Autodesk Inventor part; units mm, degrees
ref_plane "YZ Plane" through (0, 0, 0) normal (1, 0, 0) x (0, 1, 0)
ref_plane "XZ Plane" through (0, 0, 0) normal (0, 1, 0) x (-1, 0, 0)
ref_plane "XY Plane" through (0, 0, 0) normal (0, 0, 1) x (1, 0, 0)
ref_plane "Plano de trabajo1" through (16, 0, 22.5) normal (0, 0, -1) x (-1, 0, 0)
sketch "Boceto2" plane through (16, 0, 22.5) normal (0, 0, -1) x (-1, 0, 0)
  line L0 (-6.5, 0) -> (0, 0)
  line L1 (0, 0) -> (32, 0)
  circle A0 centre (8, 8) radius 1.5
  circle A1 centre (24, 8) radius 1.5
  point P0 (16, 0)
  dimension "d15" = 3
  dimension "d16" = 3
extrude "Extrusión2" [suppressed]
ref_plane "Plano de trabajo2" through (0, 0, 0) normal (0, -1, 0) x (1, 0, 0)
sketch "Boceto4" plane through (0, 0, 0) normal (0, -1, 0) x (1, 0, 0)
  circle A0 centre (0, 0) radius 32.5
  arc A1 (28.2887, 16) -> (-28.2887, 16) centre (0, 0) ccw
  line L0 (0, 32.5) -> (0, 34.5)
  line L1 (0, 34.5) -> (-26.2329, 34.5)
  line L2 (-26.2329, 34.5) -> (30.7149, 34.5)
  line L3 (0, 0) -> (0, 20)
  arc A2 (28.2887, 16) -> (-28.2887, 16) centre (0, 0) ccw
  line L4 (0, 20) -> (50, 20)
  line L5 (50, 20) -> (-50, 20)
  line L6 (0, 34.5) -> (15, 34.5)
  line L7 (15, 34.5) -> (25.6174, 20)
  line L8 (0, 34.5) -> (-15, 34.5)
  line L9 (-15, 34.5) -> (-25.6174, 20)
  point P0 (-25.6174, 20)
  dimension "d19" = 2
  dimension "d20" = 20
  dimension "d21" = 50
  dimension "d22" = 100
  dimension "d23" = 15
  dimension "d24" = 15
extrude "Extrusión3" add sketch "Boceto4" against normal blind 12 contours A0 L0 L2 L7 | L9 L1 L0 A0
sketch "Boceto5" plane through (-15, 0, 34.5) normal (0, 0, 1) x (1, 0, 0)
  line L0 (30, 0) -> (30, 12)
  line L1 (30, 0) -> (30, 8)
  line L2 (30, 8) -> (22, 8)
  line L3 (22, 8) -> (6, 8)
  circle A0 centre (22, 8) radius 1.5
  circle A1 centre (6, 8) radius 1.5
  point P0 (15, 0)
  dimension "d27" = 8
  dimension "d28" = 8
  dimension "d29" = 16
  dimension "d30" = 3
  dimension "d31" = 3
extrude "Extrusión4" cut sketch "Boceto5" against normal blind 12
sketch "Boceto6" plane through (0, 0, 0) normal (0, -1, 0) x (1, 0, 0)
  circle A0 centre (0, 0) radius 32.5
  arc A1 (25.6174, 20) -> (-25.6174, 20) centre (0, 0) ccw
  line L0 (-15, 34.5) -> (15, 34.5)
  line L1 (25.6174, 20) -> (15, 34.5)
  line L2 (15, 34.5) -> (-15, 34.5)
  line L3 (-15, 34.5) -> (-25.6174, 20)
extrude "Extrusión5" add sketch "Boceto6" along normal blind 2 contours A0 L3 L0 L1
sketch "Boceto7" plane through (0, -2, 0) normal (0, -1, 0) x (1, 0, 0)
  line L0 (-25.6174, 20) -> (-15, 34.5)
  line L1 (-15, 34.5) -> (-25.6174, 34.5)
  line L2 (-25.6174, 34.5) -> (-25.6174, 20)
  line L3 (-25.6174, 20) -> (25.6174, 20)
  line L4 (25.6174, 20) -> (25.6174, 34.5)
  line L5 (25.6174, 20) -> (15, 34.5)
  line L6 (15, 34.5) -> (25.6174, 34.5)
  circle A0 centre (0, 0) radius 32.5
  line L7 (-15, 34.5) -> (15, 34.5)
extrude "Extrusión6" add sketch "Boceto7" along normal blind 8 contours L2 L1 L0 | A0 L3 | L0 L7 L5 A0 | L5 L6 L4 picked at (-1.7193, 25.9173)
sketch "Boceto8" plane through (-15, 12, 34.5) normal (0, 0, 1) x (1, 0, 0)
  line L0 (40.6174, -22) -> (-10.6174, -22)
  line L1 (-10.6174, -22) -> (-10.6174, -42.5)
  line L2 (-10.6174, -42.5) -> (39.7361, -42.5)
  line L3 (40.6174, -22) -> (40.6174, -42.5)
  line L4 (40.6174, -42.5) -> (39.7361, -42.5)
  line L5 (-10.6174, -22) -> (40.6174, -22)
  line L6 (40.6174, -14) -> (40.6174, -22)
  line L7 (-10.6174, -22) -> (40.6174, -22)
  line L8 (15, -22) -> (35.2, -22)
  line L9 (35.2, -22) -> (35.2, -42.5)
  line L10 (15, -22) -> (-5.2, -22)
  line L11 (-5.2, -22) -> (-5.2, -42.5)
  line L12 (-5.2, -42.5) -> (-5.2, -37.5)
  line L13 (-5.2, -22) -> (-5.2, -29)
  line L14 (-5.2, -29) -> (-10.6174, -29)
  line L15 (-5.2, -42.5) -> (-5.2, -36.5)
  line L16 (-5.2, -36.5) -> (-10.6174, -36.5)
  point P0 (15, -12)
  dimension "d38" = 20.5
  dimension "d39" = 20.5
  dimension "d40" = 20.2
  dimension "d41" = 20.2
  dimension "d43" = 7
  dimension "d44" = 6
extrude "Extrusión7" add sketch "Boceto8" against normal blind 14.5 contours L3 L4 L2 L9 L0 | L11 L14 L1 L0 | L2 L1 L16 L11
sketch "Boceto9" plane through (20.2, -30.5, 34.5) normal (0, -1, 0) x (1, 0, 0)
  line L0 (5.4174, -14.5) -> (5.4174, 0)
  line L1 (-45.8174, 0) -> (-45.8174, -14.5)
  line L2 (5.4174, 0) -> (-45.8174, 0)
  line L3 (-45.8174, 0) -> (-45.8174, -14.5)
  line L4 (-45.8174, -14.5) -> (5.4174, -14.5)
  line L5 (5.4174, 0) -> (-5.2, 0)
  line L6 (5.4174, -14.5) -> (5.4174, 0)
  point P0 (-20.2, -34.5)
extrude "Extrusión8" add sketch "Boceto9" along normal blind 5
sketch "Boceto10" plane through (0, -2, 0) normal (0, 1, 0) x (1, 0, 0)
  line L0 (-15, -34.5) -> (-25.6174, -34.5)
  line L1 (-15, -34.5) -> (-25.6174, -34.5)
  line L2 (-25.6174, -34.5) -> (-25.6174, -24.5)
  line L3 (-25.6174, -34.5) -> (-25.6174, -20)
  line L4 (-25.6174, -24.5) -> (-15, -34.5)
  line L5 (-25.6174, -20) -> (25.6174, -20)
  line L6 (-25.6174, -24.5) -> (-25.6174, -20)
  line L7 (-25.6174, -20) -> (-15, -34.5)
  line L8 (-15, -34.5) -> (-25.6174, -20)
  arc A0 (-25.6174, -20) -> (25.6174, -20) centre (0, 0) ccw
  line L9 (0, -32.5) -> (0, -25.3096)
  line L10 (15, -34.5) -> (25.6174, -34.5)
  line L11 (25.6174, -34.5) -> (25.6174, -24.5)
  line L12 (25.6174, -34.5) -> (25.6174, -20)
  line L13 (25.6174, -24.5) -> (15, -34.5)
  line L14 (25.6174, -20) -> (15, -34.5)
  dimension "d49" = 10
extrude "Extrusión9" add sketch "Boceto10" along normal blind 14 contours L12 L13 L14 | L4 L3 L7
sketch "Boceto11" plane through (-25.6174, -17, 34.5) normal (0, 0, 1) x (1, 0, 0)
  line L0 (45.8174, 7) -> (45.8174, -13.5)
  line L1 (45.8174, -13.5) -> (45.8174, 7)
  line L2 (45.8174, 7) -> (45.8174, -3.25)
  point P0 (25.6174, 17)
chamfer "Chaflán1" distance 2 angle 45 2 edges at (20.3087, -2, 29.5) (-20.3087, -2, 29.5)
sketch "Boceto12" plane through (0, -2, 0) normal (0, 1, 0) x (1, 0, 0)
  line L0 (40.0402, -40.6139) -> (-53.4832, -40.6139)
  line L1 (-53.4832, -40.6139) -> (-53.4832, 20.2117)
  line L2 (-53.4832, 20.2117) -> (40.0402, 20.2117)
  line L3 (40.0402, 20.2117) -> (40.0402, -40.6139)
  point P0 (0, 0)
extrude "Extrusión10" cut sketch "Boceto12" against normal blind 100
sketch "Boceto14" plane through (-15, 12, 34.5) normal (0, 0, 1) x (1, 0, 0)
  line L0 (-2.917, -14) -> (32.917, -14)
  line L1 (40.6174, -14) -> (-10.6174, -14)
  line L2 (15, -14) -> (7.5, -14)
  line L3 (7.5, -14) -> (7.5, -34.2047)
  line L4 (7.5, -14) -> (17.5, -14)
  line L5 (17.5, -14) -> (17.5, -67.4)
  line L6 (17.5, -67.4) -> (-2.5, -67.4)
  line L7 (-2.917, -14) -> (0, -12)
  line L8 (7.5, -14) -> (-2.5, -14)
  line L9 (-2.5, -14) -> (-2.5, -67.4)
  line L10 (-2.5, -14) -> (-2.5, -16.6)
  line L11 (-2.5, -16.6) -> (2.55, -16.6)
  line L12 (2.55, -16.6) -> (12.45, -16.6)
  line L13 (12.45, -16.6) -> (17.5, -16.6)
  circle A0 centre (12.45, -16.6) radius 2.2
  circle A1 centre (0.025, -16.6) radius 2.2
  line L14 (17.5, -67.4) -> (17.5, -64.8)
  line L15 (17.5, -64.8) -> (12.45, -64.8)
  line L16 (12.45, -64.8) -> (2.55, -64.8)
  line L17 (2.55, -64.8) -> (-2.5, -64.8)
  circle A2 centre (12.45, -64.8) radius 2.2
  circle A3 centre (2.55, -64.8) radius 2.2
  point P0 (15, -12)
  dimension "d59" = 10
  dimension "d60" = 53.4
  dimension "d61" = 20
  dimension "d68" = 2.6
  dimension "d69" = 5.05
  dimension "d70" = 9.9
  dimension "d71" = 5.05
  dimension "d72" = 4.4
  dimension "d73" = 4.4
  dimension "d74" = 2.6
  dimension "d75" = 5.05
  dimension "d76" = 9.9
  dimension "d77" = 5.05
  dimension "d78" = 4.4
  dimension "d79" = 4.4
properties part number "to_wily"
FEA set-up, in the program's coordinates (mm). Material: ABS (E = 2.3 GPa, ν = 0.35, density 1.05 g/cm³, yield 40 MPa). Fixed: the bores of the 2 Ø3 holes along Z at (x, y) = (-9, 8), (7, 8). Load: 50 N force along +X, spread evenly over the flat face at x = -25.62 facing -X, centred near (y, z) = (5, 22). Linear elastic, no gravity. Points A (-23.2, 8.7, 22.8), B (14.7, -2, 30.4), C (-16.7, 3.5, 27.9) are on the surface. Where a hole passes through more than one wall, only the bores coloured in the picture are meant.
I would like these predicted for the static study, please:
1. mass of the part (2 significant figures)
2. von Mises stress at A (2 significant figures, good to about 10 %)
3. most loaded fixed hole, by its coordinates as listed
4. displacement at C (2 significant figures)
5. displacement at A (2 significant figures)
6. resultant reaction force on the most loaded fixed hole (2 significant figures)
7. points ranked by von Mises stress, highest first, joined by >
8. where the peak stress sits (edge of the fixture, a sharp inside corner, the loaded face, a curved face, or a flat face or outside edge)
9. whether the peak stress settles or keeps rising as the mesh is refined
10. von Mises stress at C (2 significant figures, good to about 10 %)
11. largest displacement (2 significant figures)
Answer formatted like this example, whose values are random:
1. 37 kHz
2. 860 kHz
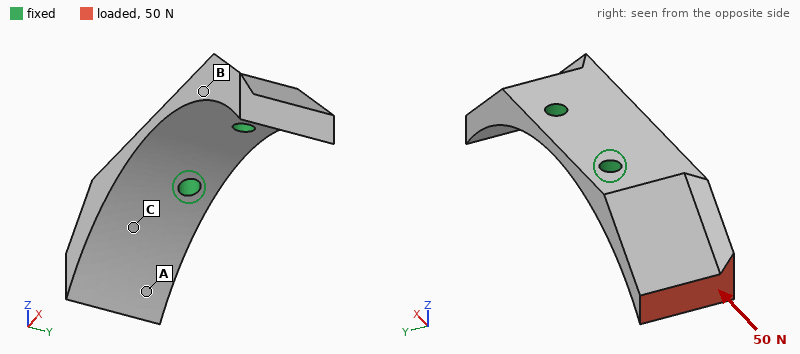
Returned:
1. 2.8 g
2. 5.5 MPa
3. (-9, 8)
4. 0.16 mm
5. 0.44 mm
6. 48 N
7. C > A > B
8. edge of the fixture
9. keeps rising
10. 11 MPa
11. 0.64 mm
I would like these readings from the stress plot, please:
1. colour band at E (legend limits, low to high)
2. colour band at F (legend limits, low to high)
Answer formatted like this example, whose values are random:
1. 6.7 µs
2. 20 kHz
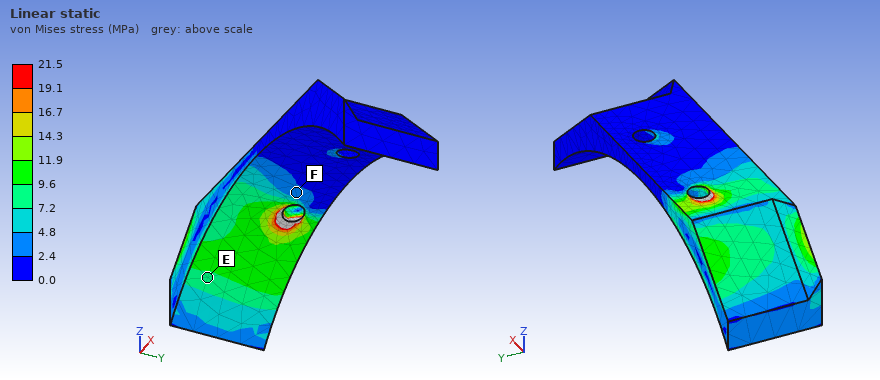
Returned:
1. 7.2 to 9.6 MPa
2. 2.4 to 4.8 MPa
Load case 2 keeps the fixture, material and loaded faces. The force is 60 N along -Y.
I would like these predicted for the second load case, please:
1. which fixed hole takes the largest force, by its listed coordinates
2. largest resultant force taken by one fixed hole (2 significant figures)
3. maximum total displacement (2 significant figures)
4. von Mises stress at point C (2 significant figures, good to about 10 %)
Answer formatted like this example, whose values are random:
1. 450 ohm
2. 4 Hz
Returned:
1. (-9, 8)
2. 100 N
3. 0.41 mm
4. 5.8 MPa
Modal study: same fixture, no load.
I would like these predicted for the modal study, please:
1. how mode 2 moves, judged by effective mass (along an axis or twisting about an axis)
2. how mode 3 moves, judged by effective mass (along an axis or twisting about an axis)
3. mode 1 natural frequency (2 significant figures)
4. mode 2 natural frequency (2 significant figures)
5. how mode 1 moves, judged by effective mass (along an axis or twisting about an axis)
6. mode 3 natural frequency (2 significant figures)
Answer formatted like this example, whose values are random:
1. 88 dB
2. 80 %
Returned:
1. along Z
2. along Y
3. 1700 Hz
4. 2400 Hz
5. along Z
6. 3000 Hz
